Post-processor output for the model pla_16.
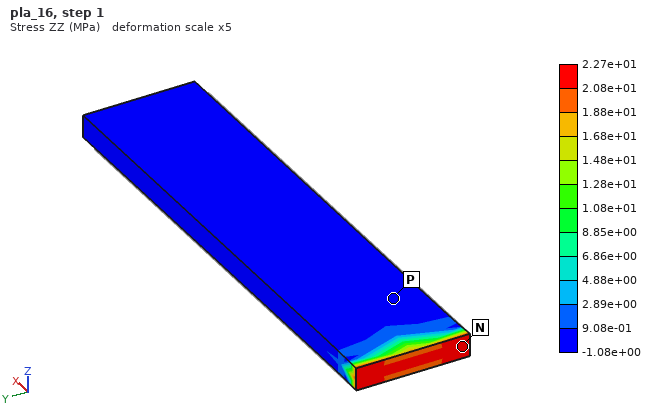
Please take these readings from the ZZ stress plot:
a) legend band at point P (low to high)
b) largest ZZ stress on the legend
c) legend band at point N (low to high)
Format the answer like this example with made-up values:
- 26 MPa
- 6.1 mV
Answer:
- -1.08e+00 to 9.08e-01 MPa
- 2.27e+01 MPa
- 2.08e+01 to 2.27e+01 MPa
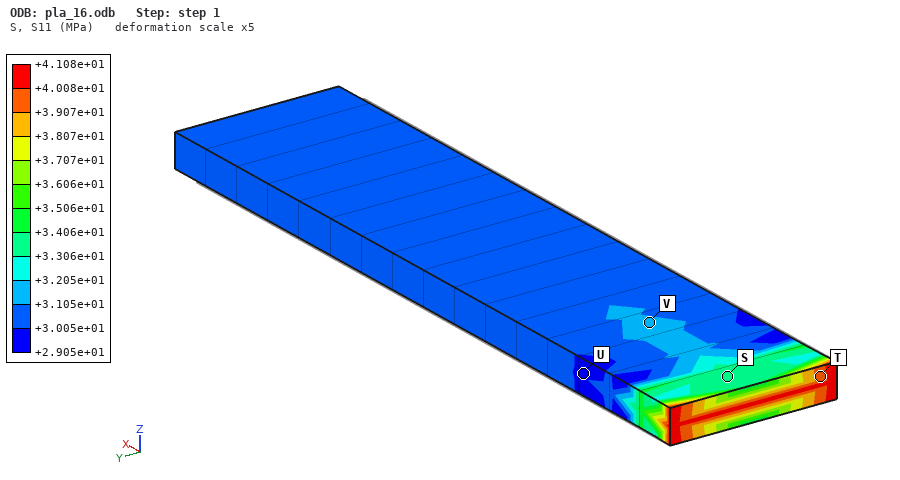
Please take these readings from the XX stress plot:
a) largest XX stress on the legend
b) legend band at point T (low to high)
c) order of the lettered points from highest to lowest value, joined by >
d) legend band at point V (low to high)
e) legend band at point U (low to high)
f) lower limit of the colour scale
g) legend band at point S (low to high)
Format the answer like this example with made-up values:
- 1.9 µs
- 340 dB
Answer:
- +4.108e+01 MPa
- +3.907e+01 to +4.008e+01 MPa
- T > S > V > U
- +3.105e+01 to +3.205e+01 MPa
- +2.905e+01 to +3.005e+01 MPa
- +2.905e+01 MPa
- +3.306e+01 to +3.406e+01 MPa
